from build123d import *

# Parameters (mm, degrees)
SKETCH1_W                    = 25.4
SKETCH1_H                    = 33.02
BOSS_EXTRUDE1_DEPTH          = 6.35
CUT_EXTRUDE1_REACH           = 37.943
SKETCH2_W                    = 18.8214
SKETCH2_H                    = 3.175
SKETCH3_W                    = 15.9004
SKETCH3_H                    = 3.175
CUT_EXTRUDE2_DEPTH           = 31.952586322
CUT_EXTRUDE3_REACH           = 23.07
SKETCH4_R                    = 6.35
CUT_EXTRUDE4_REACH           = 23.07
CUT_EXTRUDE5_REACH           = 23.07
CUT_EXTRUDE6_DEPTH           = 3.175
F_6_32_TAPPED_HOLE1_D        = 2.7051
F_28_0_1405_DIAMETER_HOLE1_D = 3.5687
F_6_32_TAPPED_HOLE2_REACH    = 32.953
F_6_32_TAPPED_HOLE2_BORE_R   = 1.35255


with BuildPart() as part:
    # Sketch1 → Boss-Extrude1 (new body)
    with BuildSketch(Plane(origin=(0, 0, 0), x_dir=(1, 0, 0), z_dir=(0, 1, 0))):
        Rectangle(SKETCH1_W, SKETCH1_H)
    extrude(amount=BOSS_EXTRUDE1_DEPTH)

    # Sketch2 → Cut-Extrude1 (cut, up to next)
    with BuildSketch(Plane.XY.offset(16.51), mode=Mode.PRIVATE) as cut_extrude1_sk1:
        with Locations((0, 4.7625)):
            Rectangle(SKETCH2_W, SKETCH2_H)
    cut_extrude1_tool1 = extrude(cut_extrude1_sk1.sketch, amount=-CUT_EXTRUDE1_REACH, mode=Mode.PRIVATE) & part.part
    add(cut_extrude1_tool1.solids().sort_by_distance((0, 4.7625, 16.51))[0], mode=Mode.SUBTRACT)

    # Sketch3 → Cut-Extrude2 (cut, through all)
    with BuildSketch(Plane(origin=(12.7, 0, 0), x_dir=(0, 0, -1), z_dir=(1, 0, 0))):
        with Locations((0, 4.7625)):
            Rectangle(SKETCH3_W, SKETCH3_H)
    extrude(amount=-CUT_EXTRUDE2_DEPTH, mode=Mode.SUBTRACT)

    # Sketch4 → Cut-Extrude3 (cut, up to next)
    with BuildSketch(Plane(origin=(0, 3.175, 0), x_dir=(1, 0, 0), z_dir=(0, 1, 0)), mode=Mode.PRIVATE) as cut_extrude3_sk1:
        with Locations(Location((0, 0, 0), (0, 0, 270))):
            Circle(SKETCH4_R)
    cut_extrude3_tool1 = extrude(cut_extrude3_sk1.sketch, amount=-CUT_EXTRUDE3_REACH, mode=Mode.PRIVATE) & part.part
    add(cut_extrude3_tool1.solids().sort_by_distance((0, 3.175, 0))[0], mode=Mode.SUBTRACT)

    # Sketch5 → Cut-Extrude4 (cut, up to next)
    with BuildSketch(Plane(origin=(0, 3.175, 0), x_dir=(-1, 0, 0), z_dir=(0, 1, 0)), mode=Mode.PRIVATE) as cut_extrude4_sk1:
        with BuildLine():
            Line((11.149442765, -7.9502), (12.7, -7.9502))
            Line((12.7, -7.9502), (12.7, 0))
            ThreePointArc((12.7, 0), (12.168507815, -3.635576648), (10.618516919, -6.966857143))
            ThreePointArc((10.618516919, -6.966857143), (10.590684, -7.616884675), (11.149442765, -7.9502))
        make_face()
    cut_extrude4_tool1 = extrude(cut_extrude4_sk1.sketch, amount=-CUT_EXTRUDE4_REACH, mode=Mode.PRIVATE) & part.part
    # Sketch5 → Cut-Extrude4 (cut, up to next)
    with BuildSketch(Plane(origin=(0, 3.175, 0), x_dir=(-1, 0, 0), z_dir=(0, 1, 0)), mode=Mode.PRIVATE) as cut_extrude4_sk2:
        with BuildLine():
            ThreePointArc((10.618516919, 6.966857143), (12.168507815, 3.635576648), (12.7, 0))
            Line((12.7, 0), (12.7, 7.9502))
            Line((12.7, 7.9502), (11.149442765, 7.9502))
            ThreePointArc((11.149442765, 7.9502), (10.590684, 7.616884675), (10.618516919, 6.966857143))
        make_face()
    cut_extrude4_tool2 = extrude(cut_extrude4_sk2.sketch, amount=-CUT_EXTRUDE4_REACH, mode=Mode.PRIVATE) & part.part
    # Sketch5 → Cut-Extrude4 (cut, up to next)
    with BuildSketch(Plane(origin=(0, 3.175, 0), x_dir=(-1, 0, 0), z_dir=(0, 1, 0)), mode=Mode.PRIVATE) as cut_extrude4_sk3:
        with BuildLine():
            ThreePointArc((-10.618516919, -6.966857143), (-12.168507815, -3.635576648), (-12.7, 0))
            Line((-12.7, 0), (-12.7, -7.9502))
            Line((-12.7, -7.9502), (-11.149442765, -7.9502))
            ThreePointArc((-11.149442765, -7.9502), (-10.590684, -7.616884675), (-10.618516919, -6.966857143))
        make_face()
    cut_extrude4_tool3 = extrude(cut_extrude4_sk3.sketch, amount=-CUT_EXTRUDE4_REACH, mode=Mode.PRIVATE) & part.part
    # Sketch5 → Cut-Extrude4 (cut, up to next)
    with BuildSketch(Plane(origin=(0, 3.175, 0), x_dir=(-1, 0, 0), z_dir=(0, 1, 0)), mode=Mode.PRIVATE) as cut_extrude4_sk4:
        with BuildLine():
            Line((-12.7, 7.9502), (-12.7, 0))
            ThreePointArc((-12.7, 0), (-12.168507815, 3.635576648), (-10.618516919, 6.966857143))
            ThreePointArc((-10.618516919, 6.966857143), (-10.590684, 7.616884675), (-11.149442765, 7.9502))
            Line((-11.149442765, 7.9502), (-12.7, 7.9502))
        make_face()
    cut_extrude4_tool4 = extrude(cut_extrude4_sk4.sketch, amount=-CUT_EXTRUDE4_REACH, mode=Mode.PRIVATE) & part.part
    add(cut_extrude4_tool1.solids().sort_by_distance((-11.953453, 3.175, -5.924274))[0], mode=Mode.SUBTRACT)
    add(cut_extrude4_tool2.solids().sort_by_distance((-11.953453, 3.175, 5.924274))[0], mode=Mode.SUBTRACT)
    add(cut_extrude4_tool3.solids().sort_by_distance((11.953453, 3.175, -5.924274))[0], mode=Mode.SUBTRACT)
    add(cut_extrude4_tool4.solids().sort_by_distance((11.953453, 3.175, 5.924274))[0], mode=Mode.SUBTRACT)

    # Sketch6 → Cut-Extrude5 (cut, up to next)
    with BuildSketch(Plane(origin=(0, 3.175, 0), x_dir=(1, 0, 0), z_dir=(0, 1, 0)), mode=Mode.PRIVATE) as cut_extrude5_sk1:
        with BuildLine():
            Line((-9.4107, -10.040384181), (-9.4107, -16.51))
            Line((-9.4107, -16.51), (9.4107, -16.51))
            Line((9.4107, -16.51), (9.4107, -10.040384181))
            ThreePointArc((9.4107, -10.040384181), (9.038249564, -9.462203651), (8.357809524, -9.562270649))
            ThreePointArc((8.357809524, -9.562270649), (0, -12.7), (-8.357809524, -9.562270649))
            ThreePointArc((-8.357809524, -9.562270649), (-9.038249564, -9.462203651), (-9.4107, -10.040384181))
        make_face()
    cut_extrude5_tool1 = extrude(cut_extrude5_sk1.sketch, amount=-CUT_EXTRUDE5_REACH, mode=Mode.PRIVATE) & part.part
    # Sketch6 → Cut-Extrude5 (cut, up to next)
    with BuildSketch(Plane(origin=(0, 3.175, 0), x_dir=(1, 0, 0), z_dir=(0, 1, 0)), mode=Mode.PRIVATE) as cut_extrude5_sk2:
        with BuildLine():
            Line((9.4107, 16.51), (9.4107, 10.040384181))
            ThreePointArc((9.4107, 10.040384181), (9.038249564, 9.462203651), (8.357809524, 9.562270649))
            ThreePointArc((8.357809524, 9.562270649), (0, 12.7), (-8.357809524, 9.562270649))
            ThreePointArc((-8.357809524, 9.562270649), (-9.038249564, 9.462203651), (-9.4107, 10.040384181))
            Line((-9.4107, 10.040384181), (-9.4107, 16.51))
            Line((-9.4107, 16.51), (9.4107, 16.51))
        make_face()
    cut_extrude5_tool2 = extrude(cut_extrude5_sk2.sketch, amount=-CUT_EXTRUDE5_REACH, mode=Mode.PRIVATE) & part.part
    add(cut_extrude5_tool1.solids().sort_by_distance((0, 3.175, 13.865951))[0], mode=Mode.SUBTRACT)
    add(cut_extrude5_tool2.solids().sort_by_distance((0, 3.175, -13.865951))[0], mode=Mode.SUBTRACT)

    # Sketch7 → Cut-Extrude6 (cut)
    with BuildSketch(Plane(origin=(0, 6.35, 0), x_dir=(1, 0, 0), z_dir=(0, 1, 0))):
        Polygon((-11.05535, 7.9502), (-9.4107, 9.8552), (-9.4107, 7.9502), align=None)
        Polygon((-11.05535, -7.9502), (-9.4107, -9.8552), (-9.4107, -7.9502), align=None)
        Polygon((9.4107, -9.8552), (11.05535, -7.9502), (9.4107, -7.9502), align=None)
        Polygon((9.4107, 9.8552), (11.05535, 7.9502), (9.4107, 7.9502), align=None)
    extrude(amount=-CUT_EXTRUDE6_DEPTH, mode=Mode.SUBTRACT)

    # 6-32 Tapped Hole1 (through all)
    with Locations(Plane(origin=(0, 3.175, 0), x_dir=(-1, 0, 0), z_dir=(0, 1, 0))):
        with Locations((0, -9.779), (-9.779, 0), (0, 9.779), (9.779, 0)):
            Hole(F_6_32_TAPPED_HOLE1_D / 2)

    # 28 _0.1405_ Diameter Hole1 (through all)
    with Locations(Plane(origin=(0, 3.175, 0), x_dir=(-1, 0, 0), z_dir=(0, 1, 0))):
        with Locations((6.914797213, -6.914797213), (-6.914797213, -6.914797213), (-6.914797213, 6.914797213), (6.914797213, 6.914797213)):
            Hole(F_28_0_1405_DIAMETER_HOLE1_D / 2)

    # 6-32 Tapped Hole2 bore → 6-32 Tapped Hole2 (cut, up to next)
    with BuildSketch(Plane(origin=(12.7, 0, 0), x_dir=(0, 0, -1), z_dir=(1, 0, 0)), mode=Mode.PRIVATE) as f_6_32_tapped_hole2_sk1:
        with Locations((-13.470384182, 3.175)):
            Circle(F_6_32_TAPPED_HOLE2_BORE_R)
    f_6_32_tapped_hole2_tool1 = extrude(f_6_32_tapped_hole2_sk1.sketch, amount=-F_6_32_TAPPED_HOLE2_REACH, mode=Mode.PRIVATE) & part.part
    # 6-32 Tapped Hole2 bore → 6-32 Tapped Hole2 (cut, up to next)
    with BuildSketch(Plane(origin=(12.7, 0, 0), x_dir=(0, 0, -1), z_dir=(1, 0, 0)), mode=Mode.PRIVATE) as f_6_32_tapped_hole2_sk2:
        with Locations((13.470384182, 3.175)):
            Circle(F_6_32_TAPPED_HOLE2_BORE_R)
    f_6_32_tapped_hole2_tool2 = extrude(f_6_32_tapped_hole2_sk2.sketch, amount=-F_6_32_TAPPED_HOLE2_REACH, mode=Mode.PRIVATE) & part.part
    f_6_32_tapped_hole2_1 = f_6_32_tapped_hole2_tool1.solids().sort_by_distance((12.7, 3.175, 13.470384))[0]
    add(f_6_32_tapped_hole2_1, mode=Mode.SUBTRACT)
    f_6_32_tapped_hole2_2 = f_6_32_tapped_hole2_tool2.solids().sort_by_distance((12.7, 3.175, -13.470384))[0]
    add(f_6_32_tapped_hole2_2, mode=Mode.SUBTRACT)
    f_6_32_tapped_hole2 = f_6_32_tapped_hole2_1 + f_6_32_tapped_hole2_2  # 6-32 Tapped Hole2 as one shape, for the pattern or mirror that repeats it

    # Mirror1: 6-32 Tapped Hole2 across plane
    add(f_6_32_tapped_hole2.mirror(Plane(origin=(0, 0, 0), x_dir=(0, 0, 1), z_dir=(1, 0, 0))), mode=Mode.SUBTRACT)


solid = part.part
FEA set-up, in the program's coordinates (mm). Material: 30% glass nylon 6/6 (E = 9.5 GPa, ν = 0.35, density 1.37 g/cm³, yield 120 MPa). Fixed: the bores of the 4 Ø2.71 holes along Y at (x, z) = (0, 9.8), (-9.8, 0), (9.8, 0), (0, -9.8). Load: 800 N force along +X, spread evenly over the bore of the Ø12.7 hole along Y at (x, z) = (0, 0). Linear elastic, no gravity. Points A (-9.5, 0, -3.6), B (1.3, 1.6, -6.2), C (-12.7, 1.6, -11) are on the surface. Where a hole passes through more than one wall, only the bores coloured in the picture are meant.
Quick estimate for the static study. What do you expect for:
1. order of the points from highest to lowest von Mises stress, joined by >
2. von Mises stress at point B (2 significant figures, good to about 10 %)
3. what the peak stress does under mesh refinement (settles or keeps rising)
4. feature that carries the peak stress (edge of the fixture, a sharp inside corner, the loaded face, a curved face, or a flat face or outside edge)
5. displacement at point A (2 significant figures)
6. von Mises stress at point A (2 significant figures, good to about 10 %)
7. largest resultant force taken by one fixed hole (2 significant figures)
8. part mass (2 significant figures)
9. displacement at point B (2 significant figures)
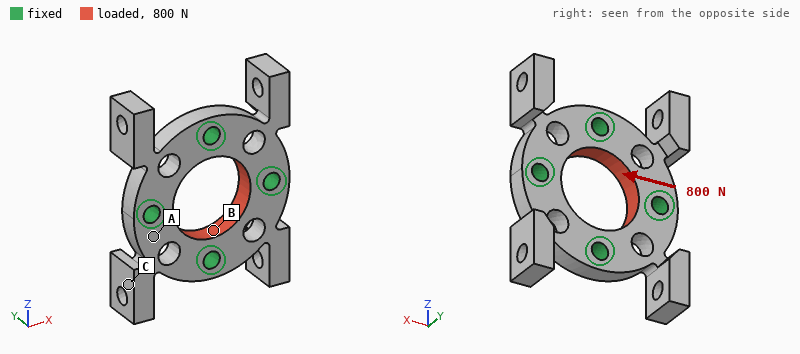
B > A > C
12 MPa
keeps rising
edge of the fixture
3.8 µm
6.5 MPa
210 N
2.2 g
7.4 µm
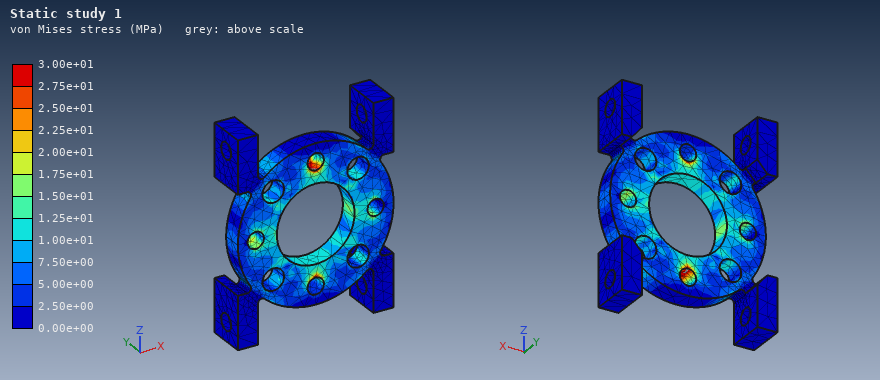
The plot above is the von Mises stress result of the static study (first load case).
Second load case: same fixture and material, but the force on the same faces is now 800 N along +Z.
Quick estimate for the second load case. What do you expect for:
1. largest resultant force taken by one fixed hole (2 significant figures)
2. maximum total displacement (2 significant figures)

210 N
10 µm
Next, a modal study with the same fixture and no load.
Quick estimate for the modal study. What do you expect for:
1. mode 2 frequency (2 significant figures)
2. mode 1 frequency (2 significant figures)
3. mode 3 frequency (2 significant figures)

5400 Hz
5400 Hz
5400 Hz
